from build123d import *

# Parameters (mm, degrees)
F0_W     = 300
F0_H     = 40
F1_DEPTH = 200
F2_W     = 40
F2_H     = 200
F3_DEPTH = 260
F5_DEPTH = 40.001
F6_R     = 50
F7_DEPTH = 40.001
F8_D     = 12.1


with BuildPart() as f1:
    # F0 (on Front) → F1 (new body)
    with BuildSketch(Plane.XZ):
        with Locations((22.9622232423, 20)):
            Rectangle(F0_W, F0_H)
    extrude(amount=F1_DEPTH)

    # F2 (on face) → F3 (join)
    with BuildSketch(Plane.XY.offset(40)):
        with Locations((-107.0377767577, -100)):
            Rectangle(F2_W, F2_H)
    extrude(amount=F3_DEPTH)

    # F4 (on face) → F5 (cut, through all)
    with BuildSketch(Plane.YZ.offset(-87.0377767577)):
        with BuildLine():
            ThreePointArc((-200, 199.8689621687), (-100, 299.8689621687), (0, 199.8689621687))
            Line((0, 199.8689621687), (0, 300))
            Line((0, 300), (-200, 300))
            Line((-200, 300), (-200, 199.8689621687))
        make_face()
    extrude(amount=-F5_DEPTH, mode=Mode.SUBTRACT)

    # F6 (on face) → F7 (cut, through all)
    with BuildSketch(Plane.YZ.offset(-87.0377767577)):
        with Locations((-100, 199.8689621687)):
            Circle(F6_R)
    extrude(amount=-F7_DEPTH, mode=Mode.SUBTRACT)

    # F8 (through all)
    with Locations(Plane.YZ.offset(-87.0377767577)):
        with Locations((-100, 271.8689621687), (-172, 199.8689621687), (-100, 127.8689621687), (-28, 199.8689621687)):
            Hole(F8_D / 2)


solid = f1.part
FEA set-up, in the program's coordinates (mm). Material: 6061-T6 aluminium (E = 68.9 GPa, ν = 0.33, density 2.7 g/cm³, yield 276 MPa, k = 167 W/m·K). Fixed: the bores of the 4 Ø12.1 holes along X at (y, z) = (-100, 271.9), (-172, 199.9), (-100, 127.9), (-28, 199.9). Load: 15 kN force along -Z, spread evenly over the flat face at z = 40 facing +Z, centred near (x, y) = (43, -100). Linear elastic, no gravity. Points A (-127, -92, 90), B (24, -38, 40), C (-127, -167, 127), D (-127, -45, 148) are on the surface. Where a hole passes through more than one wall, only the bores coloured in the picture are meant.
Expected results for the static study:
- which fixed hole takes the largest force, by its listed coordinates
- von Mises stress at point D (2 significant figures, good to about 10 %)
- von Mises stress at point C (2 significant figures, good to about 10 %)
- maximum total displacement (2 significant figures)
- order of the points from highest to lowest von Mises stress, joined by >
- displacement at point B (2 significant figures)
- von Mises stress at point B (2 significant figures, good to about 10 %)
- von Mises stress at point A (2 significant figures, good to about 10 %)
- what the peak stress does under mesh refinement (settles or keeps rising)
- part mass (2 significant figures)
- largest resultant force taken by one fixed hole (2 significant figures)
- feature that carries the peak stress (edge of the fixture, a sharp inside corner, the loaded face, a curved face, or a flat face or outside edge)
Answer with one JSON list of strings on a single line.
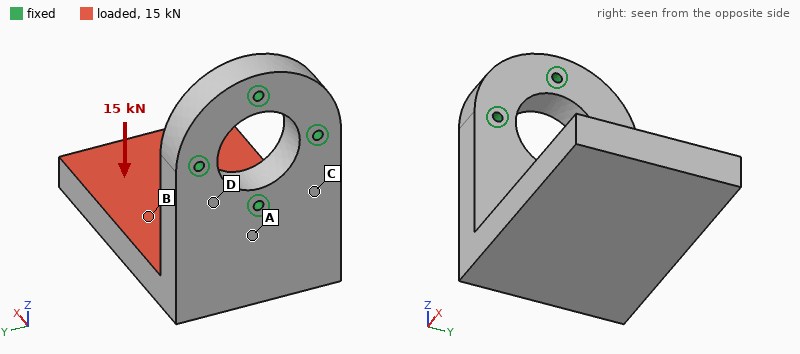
["(-100, 127.9)", "21 MPa", "27 MPa", "1.6 mm", "A > C > D > B", "0.64 mm", "12 MPa", "41 MPa", "keeps rising", "11 kg", "18 kN", "edge of the fixture"]
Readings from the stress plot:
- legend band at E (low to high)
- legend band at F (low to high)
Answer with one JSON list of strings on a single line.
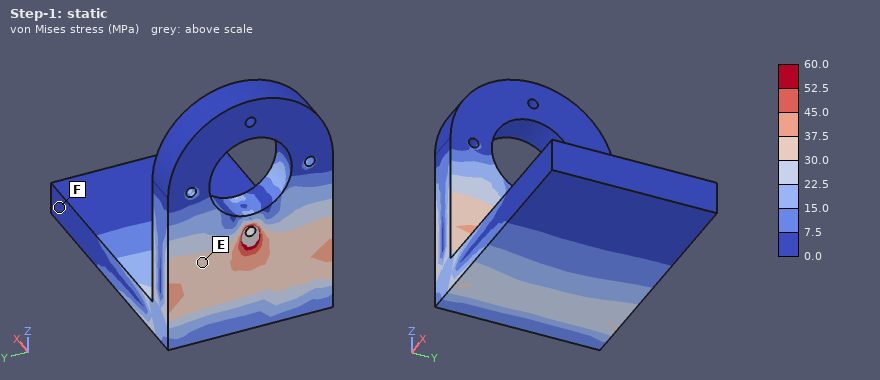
["30.0 to 37.5 MPa", "0.0 to 7.5 MPa"]
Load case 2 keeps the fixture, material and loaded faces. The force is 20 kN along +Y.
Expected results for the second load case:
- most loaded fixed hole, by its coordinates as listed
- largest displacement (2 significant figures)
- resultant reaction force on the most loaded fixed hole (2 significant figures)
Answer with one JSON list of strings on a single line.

["(-100, 127.9)", "1.1 mm", "20 kN"]
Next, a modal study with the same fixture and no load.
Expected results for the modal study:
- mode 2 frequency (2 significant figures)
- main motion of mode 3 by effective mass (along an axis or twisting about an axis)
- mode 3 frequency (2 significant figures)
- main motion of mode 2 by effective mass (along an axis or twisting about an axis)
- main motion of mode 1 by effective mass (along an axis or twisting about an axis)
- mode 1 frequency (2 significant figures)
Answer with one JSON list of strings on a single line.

["350 Hz", "along X", "830 Hz", "along Y", "along Z", "250 Hz"]
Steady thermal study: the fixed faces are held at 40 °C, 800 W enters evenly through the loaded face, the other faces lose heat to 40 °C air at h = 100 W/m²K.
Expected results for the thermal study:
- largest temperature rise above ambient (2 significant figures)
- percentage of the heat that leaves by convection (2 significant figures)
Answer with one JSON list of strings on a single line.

["62 K", "69 %"]
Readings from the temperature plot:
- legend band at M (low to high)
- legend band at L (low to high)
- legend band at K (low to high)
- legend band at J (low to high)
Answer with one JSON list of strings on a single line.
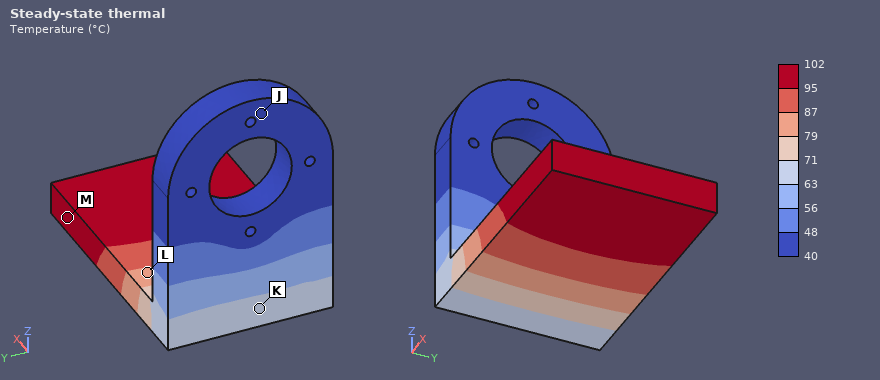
["95 to 102 °C", "79 to 87 °C", "63 to 71 °C", "40 to 48 °C"]
